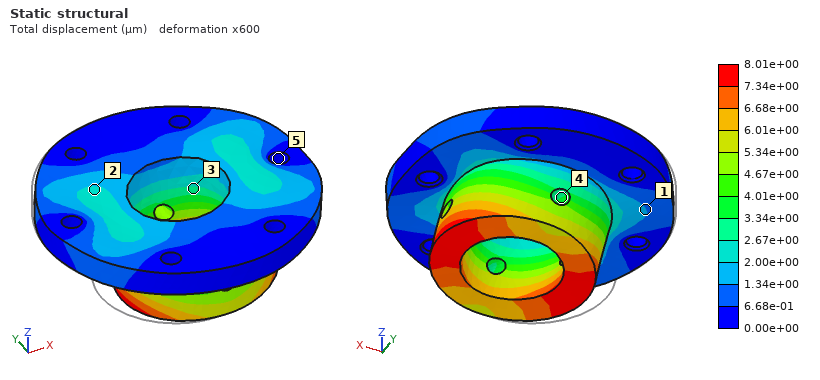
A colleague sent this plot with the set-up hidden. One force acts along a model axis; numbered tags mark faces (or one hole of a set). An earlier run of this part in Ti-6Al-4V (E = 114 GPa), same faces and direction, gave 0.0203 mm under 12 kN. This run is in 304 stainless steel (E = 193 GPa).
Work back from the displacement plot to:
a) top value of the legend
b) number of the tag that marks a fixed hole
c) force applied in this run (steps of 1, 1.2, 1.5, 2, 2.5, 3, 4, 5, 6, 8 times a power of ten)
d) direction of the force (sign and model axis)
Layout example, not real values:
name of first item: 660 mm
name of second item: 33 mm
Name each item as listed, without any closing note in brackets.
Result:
top value of the legend: 8.01e+00 µm
number of the tag that marks a fixed hole: 5
force applied in this run: 8 kN
direction of the force: +X
